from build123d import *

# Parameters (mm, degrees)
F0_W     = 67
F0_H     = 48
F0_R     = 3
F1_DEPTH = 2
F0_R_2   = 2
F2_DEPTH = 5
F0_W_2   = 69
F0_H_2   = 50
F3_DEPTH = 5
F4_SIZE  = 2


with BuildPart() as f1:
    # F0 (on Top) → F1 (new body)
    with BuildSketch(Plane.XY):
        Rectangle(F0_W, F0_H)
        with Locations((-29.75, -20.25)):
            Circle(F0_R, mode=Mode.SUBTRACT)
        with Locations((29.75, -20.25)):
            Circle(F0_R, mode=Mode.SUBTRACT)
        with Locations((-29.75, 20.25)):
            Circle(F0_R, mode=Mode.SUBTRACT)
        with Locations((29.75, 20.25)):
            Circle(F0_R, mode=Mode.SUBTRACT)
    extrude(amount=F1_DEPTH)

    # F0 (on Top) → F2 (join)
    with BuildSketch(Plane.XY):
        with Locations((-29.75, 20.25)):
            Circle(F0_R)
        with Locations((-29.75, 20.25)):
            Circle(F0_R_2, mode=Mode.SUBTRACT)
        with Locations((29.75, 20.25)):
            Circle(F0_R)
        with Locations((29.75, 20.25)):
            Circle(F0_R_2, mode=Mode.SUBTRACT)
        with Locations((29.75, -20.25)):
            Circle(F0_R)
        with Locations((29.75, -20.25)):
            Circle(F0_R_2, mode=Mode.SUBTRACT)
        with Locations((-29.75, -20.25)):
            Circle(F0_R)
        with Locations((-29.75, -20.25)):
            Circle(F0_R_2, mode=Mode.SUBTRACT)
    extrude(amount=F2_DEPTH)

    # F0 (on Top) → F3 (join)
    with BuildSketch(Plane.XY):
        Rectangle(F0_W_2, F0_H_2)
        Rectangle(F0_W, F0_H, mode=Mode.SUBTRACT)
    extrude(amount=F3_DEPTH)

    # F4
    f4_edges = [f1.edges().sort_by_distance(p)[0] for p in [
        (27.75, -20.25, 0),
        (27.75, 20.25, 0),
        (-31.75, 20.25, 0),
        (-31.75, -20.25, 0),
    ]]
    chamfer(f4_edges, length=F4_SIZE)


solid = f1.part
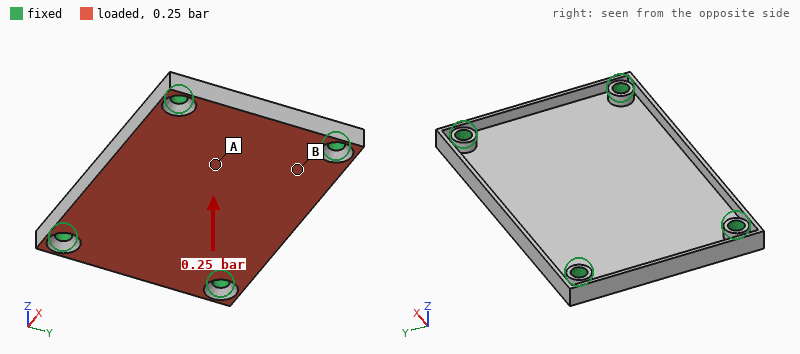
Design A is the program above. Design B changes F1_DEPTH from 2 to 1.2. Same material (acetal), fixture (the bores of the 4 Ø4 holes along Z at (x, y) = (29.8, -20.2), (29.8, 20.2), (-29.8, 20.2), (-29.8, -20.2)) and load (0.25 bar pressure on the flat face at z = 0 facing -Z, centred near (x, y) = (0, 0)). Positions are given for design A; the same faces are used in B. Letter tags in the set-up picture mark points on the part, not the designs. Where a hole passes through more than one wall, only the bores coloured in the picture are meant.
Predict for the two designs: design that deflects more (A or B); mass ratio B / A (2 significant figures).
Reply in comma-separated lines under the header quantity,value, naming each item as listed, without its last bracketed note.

quantity,value
design that deflects more,B
mass ratio B / A,0.67
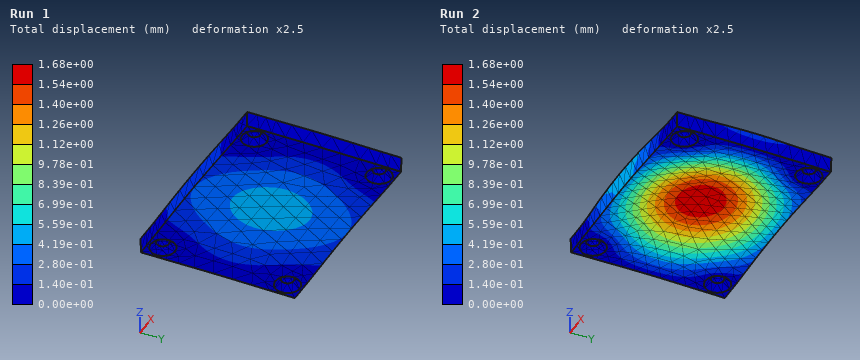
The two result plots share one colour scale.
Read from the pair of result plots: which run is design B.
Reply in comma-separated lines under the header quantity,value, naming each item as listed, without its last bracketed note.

quantity,value
which run is design B,Run 2
